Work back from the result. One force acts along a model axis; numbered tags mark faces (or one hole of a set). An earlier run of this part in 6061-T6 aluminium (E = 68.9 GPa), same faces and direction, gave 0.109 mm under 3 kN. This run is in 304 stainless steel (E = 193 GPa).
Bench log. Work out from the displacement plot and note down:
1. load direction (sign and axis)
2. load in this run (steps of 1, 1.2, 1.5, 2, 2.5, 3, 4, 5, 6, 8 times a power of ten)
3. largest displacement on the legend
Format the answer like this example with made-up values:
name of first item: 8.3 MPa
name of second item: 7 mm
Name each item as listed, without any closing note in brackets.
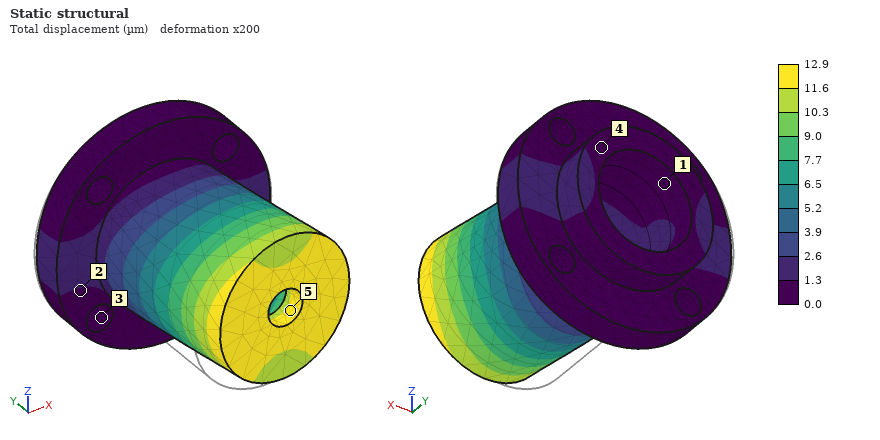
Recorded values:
load direction: +X
load in this run: 1 kN
largest displacement on the legend: 12.9 µm
